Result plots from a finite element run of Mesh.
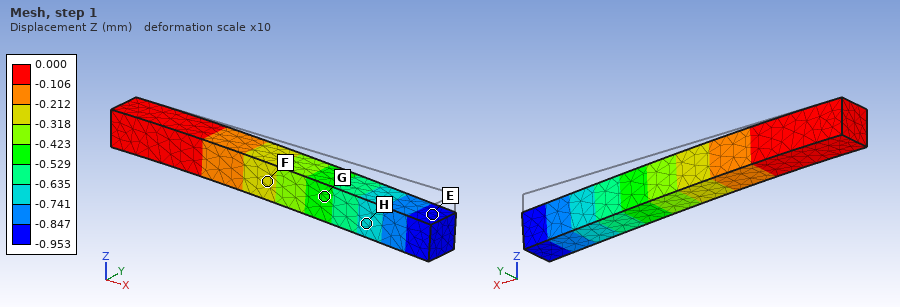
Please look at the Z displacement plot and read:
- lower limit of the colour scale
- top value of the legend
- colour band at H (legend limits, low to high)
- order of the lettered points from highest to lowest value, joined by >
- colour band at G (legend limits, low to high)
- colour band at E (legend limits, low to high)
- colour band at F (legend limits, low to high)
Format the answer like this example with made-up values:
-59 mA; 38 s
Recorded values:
-0.953 mm; 0.000 mm; -0.741 to -0.635 mm; F > G > H > E; -0.529 to -0.423 mm; -0.953 to -0.847 mm; -0.318 to -0.212 mm
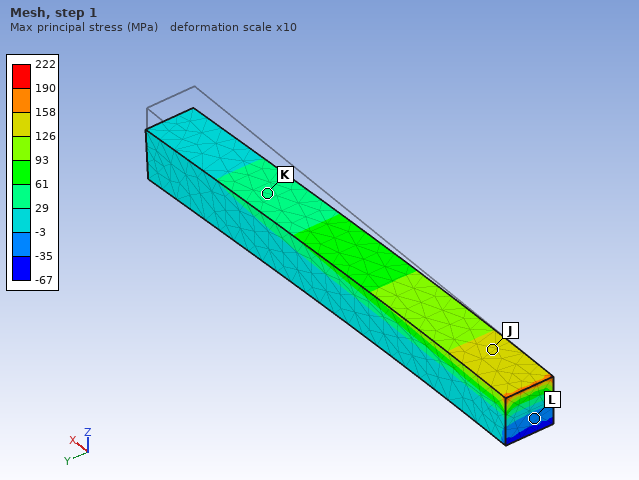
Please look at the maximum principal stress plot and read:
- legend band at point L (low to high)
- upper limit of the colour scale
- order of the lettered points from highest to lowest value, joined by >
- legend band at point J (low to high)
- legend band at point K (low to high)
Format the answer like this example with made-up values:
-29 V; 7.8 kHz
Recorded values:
-35 to -3 MPa; 222 MPa; J > K > L; 126 to 158 MPa; 29 to 61 MPa
